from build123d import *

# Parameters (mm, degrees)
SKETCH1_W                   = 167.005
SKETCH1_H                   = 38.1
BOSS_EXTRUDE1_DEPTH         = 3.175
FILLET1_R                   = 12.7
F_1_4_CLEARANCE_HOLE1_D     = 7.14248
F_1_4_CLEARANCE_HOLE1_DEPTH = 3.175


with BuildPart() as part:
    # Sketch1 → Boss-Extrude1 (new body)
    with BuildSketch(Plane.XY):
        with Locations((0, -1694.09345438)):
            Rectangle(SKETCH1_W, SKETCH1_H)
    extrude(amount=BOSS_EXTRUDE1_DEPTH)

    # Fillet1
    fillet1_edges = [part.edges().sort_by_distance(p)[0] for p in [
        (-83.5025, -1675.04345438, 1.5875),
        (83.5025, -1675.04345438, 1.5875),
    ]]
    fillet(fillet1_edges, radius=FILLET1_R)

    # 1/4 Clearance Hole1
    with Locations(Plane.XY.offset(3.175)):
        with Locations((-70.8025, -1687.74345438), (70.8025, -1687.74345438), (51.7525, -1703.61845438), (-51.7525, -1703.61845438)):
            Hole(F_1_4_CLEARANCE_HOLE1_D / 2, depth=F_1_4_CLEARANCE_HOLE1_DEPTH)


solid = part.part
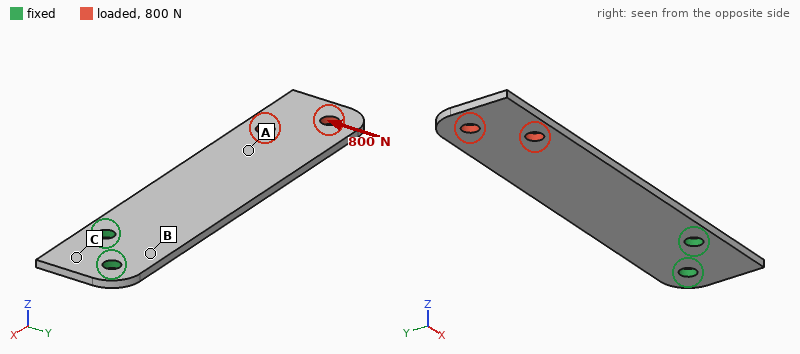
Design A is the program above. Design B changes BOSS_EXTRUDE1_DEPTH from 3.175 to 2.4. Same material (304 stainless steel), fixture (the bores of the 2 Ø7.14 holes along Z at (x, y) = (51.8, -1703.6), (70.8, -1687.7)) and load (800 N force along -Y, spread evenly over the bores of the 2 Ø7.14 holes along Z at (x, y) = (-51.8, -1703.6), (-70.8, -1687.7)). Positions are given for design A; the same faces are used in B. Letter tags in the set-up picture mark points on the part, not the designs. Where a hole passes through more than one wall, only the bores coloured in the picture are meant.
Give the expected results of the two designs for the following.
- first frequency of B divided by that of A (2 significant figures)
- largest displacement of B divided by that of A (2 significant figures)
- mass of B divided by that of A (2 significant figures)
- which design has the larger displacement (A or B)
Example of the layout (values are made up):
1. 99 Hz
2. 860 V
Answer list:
1. 0.76
2. 1.3
3. 0.76
4. B
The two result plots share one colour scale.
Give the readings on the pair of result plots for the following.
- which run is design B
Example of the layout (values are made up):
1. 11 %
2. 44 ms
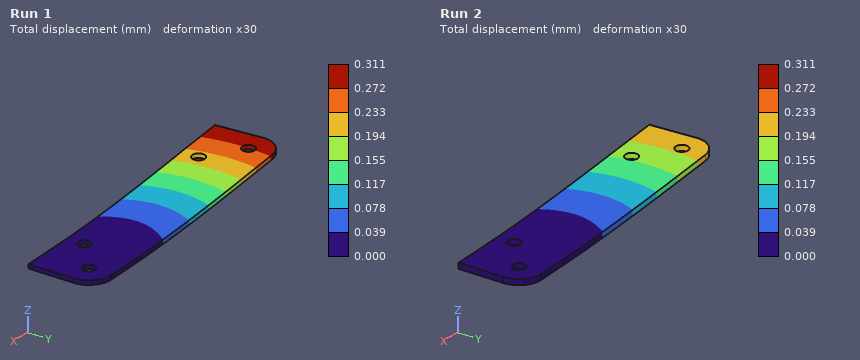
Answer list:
1. Run 1
